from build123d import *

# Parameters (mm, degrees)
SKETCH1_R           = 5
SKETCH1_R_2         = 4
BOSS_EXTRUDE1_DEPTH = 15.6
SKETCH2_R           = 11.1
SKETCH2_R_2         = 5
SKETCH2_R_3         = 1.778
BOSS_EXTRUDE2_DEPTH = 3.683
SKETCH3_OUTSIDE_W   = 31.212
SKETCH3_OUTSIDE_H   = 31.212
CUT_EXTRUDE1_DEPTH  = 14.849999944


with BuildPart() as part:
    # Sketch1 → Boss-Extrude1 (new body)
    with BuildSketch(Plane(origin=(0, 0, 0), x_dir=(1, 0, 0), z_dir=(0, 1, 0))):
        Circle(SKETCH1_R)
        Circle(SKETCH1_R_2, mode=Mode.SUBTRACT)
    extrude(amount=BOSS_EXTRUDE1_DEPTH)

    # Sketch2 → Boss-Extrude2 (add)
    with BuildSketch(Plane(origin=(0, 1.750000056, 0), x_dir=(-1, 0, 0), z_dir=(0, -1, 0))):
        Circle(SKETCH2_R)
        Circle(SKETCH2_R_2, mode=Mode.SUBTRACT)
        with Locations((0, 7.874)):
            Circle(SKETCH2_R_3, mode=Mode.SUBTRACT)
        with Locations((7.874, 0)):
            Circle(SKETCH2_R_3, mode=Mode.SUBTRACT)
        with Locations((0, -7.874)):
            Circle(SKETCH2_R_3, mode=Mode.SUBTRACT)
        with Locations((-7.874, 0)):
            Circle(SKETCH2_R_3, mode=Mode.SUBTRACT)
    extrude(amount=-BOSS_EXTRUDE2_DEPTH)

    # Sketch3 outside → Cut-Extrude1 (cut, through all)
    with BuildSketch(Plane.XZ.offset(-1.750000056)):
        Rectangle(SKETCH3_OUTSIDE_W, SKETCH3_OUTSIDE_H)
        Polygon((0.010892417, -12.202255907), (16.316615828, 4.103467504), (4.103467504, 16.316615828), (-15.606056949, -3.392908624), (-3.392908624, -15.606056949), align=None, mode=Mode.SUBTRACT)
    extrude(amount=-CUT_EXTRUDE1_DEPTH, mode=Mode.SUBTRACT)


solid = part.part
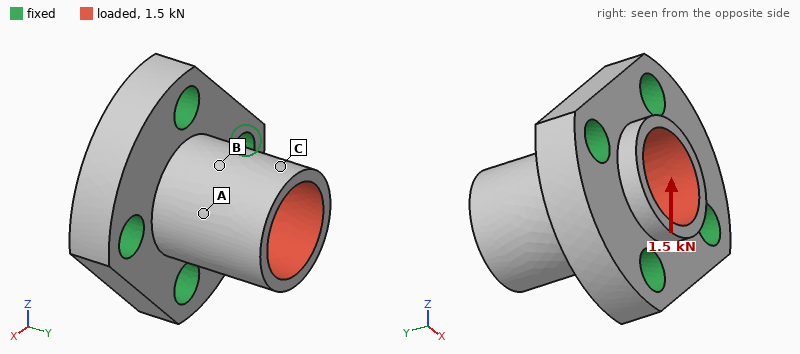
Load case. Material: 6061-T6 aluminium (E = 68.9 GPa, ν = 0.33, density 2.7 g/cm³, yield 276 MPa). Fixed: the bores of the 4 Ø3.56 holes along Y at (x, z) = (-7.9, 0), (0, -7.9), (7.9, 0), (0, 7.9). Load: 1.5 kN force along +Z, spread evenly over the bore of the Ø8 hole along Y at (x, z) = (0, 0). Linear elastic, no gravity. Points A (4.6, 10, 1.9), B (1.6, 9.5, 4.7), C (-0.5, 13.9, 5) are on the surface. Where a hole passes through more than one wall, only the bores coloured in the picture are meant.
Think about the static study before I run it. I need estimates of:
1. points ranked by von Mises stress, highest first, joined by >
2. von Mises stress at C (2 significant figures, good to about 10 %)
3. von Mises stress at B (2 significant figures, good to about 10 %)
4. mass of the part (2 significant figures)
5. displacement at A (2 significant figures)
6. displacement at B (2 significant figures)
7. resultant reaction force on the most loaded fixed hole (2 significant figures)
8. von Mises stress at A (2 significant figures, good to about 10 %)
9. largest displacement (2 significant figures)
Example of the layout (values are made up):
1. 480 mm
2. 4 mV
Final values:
1. A > B > C
2. 17 MPa
3. 34 MPa
4. 3.4 g
5. 15 µm
6. 16 µm
7. 630 N
8. 57 MPa
9. 28 µm
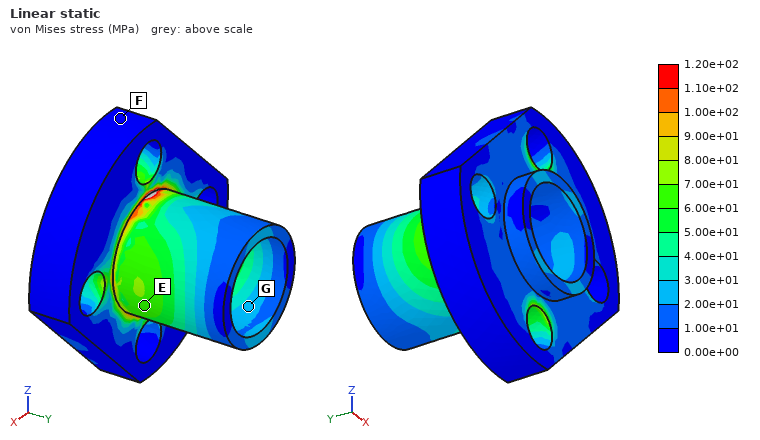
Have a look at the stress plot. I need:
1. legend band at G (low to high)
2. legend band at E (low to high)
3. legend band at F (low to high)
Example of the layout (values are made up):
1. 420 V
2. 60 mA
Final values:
1. 2.00e+01 to 3.00e+01 MPa
2. 6.00e+01 to 7.00e+01 MPa
3. 0.00e+00 to 1.00e+01 MPa
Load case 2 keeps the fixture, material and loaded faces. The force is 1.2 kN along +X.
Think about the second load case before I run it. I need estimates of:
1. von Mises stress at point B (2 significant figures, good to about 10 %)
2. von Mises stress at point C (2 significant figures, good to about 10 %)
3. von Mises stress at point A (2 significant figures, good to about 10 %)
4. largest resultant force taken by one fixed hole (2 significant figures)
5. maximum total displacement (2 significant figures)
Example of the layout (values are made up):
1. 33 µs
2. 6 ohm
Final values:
1. 49 MPa
2. 16 MPa
3. 27 MPa
4. 510 N
5. 23 µm
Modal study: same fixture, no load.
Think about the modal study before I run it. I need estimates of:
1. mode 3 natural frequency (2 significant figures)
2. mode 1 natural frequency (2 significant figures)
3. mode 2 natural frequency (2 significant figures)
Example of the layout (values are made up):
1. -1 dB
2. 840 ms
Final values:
1. 39 kHz
2. 39 kHz
3. 39 kHz
